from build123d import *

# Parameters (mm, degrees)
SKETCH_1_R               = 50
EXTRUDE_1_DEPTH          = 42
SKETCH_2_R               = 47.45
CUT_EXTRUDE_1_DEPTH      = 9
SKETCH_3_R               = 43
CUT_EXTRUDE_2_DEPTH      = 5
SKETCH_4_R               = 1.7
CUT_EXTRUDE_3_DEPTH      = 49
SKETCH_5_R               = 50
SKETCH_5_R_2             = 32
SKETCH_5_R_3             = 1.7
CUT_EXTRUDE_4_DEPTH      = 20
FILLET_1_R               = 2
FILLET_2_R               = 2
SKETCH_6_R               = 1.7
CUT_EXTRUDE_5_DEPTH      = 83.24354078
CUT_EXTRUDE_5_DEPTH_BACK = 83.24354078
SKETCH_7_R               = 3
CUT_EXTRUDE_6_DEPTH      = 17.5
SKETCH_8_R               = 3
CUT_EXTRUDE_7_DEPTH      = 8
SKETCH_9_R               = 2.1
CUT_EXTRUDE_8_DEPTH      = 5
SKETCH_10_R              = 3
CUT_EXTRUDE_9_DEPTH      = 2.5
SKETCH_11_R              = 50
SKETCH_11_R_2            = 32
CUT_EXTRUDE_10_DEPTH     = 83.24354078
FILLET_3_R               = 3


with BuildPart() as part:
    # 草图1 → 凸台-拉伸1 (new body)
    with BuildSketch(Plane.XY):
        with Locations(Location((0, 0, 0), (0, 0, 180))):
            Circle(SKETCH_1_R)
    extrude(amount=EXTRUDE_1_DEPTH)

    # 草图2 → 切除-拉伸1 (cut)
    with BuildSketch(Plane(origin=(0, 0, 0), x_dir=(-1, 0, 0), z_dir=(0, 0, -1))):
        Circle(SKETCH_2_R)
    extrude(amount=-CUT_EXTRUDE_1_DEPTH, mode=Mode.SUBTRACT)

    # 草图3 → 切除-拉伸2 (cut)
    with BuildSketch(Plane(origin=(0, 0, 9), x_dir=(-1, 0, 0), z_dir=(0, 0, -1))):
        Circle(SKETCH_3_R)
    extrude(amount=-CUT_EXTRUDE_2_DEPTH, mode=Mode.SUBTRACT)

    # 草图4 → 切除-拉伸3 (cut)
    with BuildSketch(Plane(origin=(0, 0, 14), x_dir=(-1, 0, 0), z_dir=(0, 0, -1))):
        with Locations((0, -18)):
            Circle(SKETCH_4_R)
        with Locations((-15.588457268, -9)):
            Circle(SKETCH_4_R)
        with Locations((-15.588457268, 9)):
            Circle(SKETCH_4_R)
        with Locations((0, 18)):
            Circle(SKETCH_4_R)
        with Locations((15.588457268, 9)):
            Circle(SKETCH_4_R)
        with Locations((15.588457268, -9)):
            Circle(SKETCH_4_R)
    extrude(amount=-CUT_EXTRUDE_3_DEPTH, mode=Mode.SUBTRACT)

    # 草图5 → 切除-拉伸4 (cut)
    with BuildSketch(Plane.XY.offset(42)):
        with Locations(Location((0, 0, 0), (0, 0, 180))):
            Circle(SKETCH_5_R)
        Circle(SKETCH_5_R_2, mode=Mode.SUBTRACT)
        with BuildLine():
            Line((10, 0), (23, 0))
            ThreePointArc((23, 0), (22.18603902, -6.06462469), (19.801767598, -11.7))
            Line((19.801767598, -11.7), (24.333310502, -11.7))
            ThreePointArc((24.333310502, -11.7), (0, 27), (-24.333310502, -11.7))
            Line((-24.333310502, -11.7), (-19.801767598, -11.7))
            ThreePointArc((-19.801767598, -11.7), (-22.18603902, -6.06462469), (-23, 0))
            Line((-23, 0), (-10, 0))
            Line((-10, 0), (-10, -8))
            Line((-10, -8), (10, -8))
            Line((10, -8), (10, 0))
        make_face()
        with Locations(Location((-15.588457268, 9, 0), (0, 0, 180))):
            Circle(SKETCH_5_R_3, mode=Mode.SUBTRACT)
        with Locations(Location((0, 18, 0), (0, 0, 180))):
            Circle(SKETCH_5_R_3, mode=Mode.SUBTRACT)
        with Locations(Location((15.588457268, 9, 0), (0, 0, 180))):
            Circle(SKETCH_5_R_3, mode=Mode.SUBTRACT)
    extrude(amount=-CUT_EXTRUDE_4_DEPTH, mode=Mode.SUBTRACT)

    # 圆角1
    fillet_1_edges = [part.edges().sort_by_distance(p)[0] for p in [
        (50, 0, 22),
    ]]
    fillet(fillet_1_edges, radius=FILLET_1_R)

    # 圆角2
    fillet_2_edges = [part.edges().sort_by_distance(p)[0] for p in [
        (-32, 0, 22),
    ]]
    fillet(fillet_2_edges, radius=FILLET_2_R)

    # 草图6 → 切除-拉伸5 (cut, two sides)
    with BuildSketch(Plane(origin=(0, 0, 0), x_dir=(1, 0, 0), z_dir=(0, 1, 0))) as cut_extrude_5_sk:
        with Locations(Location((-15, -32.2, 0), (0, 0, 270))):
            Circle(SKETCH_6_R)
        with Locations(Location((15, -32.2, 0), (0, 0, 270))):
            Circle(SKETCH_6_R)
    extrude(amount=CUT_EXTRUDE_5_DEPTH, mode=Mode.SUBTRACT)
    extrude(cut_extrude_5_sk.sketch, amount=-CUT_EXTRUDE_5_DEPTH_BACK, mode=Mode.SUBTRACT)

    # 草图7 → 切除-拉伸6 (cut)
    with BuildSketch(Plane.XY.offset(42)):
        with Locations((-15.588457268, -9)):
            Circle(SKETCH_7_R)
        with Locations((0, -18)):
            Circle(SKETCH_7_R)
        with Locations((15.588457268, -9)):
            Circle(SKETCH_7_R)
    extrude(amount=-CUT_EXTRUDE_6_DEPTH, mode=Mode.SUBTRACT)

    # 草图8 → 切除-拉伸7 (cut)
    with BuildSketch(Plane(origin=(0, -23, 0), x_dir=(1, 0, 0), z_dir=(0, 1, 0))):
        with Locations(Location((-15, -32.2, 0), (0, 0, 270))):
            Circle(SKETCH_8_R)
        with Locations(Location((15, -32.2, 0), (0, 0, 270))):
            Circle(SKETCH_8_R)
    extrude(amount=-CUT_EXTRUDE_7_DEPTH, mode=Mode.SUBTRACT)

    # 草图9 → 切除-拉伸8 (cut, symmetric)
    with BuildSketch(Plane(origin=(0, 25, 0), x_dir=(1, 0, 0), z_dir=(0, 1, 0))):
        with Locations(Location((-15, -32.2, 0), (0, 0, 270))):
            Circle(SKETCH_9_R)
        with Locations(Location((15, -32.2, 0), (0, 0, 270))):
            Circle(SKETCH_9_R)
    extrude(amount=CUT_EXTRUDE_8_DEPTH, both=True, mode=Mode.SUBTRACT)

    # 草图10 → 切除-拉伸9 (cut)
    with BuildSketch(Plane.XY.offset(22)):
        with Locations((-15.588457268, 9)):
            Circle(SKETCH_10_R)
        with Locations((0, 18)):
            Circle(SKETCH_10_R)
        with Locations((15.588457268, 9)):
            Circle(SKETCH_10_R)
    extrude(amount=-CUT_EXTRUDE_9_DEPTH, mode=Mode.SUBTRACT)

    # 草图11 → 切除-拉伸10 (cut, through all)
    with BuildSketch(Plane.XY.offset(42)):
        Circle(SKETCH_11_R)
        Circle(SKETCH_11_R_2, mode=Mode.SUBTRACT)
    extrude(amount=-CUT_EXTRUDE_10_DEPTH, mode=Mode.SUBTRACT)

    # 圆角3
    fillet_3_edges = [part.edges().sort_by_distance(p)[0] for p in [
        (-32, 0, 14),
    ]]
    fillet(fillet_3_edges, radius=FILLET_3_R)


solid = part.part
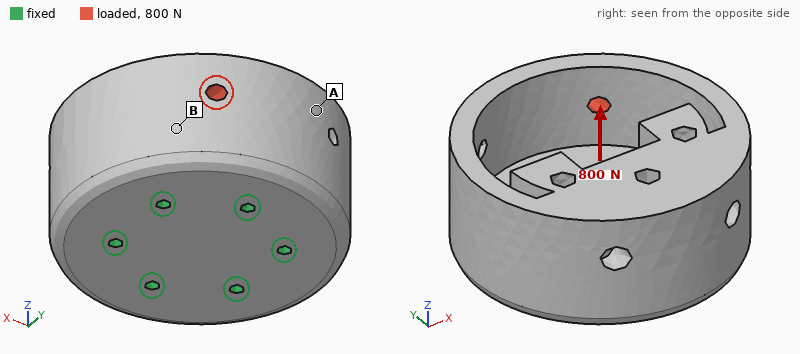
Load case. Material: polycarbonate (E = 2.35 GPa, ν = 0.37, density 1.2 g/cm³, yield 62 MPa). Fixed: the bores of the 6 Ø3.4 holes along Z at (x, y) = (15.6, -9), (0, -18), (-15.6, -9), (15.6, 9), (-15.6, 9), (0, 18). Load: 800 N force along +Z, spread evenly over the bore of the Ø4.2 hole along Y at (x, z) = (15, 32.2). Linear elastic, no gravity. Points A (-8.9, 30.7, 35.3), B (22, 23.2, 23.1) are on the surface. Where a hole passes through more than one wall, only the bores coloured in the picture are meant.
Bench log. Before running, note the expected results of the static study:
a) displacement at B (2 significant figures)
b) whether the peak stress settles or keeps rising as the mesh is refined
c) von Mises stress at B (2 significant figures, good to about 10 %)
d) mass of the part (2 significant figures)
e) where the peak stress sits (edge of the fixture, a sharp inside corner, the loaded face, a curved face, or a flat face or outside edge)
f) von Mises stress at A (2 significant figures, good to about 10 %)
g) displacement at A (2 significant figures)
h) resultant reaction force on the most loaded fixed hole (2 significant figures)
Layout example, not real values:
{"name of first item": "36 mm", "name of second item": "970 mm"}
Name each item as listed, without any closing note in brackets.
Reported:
{"displacement at B": "0.23 mm", "whether the peak stress settles or keeps rising as the mesh is refined": "keeps rising", "von Mises stress at B": "7.5 MPa", "mass of the part": "70 g", "where the peak stress sits": "edge of the fixture", "von Mises stress at A": "2.7 MPa", "displacement at A": "0.13 mm", "resultant reaction force on the most loaded fixed hole": "500 N"}
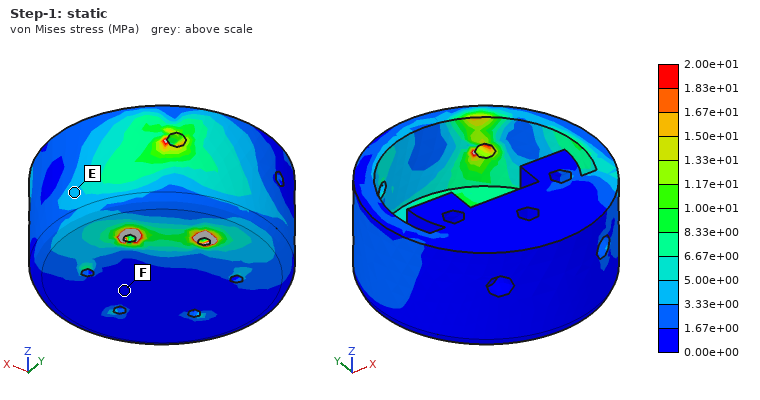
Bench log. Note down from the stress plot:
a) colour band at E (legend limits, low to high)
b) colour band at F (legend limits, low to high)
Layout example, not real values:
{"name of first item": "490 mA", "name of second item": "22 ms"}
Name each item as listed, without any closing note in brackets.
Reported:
{"colour band at E": "3.33e+00 to 5.00e+00 MPa", "colour band at F": "0.00e+00 to 1.67e+00 MPa"}
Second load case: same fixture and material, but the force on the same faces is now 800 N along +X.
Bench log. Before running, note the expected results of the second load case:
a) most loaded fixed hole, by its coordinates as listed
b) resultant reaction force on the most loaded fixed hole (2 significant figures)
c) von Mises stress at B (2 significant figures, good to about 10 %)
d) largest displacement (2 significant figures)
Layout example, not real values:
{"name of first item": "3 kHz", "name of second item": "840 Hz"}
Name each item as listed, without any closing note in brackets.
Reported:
{"most loaded fixed hole, by its coordinates as listed": "(0, 18)", "resultant reaction force on the most loaded fixed hole": "490 N", "von Mises stress at B": "9.7 MPa", "largest displacement": "0.42 mm"}
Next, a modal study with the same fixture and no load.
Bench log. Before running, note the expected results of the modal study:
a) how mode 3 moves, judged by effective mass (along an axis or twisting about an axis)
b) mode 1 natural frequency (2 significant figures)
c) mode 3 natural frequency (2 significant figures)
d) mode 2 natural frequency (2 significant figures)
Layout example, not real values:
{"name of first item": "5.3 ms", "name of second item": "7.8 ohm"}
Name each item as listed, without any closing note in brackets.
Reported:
{"how mode 3 moves, judged by effective mass": "along Y", "mode 1 natural frequency": "2800 Hz", "mode 3 natural frequency": "3300 Hz", "mode 2 natural frequency": "2800 Hz"}
